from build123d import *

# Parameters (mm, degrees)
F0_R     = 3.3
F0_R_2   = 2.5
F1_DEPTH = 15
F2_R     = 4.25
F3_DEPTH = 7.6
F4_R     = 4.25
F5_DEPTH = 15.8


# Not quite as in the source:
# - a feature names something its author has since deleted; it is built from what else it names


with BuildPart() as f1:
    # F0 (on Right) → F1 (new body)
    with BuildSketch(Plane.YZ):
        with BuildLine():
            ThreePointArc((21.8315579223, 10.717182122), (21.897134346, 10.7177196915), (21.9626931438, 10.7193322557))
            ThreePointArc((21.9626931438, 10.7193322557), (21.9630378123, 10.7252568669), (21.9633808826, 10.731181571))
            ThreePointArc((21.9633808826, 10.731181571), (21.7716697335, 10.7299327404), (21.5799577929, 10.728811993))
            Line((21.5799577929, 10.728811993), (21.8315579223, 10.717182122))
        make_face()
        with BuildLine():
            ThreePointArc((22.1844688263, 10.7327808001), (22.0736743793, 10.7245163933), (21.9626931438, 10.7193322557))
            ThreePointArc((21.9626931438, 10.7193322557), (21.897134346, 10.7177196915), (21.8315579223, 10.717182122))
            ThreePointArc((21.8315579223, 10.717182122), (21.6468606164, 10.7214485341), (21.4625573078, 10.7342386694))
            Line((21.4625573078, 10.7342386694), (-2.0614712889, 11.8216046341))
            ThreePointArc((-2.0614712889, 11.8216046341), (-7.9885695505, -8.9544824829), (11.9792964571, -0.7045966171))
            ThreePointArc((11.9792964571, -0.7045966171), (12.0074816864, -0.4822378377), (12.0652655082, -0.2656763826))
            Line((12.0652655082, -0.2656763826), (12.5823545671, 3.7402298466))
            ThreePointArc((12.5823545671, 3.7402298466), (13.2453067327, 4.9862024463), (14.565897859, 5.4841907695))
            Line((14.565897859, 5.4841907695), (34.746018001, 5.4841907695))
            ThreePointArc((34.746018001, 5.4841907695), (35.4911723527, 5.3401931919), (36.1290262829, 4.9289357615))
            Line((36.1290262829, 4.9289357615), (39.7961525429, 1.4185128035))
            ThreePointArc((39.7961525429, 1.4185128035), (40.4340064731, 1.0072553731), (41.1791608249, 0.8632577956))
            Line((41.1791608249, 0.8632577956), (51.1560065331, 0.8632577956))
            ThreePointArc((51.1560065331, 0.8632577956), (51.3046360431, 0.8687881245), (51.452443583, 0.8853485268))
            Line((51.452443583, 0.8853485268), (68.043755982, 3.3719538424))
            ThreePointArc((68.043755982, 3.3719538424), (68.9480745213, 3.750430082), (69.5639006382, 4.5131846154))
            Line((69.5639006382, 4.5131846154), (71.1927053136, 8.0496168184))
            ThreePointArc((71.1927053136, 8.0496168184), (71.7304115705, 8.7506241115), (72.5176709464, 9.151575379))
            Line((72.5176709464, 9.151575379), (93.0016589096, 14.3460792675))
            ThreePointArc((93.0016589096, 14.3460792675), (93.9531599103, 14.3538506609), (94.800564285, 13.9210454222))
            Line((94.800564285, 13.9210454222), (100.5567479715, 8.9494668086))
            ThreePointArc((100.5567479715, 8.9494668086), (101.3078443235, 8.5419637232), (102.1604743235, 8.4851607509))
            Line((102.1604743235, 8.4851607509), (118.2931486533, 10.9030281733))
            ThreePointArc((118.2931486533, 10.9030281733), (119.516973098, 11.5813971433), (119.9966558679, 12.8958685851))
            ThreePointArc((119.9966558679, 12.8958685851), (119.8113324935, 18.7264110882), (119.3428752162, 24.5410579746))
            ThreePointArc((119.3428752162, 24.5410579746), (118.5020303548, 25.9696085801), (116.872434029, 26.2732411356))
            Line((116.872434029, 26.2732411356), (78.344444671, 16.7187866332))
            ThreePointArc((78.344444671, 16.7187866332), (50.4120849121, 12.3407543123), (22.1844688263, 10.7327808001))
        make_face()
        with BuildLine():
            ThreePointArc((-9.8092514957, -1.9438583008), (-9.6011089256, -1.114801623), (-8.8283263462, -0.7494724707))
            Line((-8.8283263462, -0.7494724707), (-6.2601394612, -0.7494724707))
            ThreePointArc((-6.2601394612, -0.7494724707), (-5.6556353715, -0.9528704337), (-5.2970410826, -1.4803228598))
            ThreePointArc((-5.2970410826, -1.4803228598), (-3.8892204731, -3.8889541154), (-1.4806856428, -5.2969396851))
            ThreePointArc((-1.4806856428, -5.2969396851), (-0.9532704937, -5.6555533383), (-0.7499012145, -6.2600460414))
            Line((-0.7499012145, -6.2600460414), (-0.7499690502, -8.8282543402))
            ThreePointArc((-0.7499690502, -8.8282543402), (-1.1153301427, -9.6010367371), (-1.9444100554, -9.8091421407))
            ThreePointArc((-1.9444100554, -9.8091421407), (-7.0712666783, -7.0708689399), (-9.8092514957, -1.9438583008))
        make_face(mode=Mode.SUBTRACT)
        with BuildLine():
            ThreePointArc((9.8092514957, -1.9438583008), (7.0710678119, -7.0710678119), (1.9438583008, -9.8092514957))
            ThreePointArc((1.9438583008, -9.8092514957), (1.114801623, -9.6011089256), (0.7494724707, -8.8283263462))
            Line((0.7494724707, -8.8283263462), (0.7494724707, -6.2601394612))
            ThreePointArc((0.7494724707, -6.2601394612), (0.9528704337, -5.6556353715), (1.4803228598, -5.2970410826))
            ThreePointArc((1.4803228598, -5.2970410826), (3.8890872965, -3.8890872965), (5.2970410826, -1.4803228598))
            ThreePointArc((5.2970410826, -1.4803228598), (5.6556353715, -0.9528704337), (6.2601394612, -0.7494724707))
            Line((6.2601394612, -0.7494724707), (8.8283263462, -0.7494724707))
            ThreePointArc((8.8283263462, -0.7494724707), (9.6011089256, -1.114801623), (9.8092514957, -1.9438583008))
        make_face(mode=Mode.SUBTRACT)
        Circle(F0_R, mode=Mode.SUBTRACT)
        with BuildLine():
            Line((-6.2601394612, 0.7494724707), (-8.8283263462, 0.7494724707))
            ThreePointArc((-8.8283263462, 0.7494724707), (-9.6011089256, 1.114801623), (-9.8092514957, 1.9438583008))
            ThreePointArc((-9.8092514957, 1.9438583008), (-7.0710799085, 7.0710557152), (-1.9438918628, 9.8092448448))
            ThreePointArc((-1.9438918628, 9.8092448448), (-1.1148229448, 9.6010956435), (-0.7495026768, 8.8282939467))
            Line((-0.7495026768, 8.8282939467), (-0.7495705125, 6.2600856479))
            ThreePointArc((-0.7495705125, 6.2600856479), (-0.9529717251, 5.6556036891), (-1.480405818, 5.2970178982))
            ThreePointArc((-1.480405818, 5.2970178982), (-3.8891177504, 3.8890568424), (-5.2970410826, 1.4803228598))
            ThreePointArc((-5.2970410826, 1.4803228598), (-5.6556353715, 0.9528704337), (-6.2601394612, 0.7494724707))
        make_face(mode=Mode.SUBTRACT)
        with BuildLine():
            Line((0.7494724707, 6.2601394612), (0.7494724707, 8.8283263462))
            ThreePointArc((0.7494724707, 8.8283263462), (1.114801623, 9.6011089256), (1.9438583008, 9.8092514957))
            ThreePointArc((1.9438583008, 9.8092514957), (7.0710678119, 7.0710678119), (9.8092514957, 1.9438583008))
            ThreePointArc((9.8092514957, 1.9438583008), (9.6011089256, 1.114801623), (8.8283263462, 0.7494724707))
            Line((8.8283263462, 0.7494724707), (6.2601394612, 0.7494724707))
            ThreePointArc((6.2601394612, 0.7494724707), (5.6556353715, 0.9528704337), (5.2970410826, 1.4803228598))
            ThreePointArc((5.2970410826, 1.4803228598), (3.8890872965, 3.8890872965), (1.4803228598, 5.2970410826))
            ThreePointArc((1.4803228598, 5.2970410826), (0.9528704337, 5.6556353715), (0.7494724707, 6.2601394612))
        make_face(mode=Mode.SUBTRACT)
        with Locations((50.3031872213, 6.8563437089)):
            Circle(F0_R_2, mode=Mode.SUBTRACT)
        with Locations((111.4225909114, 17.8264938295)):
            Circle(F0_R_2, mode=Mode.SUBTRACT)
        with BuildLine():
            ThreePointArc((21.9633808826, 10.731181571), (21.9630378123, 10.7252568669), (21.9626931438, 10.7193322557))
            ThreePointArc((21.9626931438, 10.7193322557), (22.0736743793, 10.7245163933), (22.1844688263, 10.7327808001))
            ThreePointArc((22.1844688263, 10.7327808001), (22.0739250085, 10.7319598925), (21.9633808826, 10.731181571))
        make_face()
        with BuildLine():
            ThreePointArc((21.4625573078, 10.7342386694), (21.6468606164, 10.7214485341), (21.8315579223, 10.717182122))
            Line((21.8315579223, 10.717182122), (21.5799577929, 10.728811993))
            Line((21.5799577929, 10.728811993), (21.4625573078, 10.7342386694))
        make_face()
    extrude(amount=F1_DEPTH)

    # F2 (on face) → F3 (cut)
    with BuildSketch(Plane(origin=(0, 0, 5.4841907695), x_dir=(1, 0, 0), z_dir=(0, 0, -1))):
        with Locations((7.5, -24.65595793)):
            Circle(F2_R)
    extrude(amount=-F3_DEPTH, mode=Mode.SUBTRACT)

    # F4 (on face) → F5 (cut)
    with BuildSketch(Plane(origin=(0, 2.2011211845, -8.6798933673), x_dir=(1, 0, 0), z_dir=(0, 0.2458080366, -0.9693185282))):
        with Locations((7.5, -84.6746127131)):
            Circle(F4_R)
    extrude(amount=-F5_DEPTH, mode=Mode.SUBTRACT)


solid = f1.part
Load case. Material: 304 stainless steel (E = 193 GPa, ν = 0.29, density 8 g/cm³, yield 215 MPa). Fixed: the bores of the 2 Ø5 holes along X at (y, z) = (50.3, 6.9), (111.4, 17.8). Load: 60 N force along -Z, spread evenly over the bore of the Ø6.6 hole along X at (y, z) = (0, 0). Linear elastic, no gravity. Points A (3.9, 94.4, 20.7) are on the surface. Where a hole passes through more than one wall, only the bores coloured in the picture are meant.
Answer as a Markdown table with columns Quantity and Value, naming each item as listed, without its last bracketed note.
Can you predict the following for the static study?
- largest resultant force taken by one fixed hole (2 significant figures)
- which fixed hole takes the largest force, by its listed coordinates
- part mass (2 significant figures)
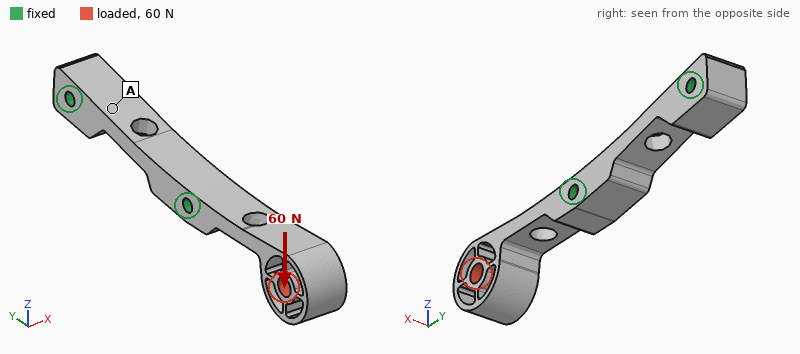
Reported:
| Quantity | Value |
|---|---|
| largest resultant force taken by one fixed hole | 65 N |
| which fixed hole takes the largest force, by its listed coordinates | (50.3, 6.9) |
| part mass | 140 g |
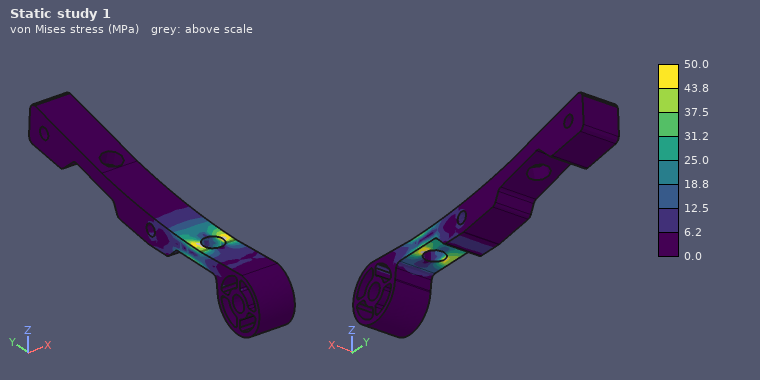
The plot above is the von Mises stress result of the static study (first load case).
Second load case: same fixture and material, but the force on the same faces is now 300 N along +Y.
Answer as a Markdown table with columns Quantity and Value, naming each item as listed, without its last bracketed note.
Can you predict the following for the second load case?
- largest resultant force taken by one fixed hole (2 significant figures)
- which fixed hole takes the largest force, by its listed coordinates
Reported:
| Quantity | Value |
|---|---|
| largest resultant force taken by one fixed hole | 300 N |
| which fixed hole takes the largest force, by its listed coordinates | (50.3, 6.9) |
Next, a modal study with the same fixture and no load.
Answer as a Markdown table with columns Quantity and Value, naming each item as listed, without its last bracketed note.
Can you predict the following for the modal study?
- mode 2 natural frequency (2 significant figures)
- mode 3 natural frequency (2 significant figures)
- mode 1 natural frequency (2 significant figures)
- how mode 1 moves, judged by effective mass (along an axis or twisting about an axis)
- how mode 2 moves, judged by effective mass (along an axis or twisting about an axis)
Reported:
| Quantity | Value |
|---|---|
| mode 2 natural frequency | 2100 Hz |
| mode 3 natural frequency | 4600 Hz |
| mode 1 natural frequency | 970 Hz |
| how mode 1 moves, judged by effective mass | along Z |
| how mode 2 moves, judged by effective mass | along X |
